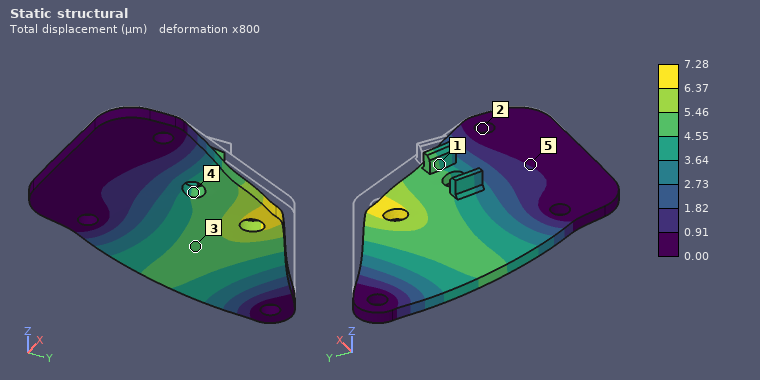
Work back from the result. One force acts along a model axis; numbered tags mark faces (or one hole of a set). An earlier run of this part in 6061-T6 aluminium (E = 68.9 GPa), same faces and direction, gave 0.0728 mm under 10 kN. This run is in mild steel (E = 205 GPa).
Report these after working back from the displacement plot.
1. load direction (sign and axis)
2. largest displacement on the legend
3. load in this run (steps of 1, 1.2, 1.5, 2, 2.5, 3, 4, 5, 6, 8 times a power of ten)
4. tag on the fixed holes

-X
7.28 µm
3 kN
2
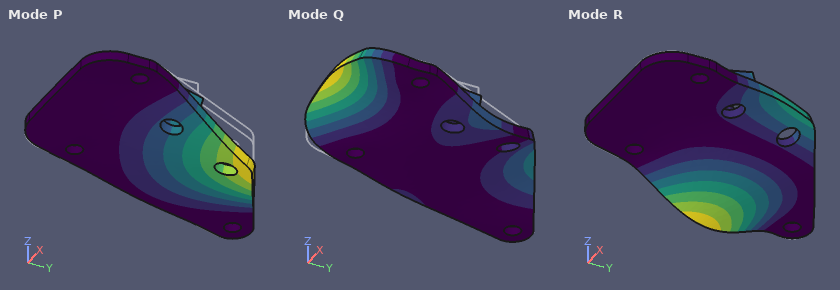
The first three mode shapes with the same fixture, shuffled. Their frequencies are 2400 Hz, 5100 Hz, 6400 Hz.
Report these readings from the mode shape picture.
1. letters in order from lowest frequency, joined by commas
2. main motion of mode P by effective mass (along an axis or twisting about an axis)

P, R, Q
along Z
